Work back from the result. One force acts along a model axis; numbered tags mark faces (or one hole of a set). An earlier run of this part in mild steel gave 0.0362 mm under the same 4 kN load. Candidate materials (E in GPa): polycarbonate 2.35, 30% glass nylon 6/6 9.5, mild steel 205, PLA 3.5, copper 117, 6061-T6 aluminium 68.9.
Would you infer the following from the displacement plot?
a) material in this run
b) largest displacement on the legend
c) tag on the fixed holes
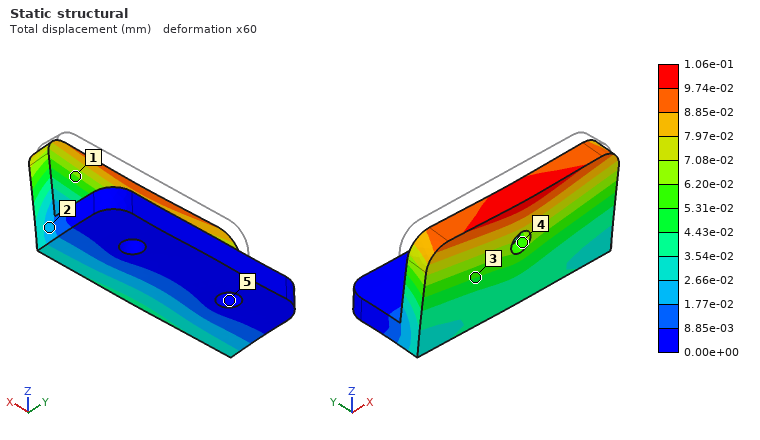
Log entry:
6061-T6 aluminium
1.06e-01 mm
5
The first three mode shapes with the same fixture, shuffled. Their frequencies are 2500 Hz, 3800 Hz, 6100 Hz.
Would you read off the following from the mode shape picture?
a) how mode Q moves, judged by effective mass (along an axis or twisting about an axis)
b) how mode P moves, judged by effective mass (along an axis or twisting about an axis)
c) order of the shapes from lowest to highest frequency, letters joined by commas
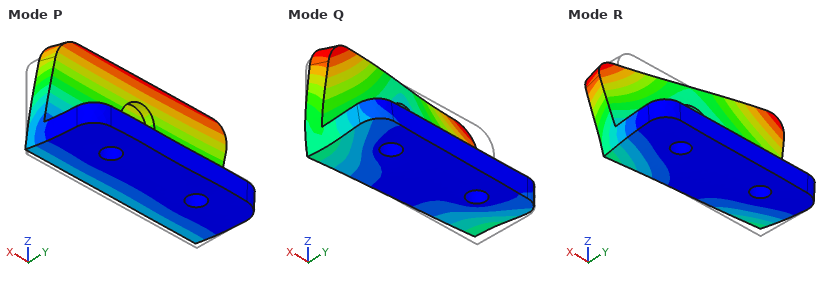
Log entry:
along X
along Y
P, R, Q
